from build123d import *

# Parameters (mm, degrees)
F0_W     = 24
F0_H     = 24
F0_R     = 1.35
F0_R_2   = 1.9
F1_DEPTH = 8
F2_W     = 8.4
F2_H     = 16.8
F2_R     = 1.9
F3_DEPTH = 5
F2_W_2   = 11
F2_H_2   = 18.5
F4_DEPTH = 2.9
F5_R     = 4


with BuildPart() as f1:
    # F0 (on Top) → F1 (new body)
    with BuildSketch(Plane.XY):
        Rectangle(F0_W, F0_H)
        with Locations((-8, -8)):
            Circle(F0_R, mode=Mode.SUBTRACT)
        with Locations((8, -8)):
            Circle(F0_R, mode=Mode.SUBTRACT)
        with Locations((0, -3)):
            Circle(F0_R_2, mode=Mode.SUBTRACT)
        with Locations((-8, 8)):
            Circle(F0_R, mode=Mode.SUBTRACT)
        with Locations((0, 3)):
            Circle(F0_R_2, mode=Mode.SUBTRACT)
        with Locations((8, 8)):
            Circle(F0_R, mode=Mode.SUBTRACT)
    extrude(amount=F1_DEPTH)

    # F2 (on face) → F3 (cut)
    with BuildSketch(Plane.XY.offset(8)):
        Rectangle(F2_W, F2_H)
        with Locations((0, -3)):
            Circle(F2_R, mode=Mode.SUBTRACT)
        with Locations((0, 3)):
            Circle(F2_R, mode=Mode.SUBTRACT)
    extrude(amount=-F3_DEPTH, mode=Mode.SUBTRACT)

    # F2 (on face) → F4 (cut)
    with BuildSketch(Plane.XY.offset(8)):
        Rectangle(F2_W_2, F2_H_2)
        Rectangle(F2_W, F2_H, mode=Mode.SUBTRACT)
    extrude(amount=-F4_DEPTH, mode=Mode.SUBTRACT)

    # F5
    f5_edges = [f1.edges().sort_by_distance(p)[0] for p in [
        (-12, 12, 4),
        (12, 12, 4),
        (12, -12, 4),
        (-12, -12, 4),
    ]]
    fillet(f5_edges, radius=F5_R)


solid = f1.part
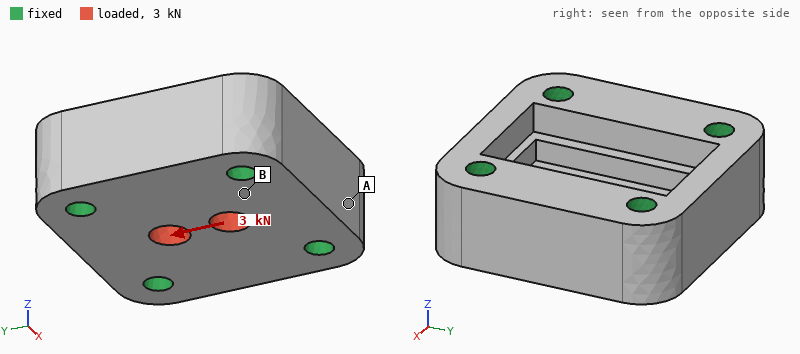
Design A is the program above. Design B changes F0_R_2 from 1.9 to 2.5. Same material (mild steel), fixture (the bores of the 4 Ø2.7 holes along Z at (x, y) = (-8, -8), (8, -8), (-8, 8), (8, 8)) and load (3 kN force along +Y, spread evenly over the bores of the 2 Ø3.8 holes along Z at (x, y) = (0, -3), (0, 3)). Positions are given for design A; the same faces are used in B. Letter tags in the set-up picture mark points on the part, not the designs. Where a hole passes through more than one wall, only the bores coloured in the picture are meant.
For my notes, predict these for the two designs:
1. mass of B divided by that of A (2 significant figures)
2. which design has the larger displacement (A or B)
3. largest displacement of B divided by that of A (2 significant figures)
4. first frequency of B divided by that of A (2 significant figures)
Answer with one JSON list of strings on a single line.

["0.99", "B", "1.5", "1.0"]
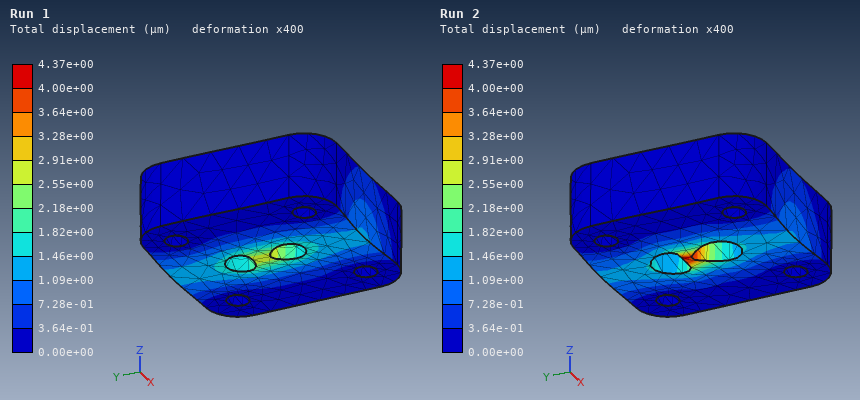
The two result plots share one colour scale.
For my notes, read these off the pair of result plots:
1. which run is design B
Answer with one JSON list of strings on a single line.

["Run 2"]
